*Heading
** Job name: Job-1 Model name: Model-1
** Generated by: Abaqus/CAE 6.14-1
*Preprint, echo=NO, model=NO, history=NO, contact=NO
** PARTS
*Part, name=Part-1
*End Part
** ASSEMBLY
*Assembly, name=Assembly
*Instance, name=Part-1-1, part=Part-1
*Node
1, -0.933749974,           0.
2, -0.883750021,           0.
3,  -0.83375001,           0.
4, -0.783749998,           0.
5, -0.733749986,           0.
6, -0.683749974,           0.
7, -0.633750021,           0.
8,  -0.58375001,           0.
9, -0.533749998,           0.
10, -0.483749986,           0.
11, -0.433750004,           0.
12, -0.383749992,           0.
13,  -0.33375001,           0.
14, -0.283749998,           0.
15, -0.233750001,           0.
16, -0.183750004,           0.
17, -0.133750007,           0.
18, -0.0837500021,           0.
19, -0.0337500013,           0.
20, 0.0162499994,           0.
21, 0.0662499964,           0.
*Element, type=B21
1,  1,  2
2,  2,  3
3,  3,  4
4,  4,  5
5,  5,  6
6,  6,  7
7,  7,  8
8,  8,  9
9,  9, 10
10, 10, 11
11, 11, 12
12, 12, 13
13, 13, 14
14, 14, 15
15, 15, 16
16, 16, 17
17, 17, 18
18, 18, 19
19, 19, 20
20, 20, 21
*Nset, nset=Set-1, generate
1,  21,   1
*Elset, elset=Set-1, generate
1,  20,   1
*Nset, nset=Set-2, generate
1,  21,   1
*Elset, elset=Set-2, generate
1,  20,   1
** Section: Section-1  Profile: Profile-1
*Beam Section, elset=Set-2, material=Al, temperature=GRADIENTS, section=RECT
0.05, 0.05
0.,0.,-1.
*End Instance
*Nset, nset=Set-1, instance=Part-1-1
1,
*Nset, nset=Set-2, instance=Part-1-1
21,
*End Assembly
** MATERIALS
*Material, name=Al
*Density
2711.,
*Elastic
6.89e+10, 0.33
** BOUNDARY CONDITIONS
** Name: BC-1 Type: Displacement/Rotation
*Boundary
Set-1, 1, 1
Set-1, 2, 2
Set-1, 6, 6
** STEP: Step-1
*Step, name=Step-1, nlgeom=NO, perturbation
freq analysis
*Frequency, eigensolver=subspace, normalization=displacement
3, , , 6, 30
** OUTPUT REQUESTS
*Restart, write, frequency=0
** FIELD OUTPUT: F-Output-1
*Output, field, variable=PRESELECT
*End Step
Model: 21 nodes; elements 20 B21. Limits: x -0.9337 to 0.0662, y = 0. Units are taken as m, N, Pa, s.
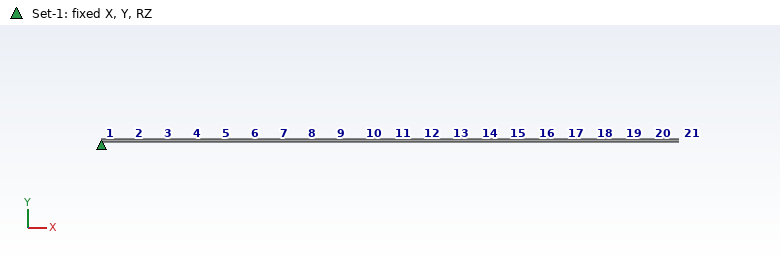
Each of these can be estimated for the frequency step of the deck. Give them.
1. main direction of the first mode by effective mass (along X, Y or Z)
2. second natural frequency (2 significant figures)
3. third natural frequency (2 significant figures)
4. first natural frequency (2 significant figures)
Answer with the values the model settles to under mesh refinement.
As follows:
along Y
250 Hz
690 Hz
41 Hz
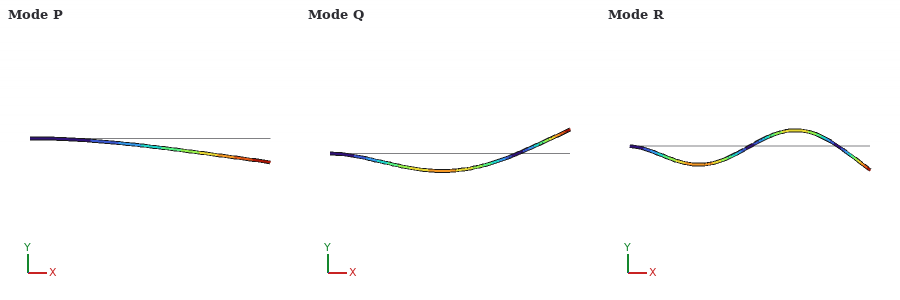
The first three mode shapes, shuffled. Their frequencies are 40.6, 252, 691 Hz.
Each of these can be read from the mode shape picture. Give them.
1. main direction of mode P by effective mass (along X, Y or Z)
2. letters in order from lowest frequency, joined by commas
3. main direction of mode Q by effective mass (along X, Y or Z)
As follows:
along Y
P, Q, R
along Y
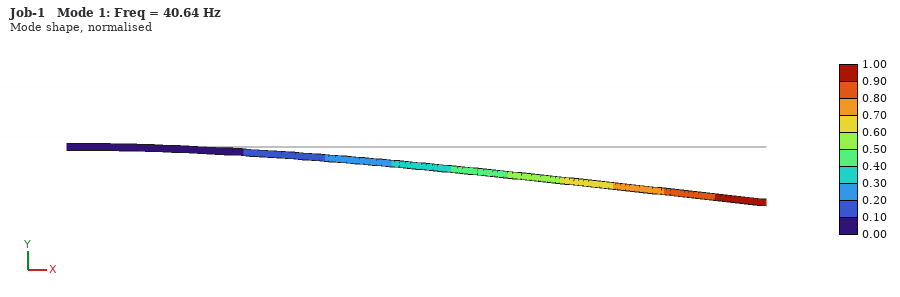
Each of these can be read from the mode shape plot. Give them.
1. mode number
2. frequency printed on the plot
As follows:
1
40.64 Hz
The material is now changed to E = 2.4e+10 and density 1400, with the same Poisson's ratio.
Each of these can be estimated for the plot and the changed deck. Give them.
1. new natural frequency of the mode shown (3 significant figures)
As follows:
33.4 Hz
